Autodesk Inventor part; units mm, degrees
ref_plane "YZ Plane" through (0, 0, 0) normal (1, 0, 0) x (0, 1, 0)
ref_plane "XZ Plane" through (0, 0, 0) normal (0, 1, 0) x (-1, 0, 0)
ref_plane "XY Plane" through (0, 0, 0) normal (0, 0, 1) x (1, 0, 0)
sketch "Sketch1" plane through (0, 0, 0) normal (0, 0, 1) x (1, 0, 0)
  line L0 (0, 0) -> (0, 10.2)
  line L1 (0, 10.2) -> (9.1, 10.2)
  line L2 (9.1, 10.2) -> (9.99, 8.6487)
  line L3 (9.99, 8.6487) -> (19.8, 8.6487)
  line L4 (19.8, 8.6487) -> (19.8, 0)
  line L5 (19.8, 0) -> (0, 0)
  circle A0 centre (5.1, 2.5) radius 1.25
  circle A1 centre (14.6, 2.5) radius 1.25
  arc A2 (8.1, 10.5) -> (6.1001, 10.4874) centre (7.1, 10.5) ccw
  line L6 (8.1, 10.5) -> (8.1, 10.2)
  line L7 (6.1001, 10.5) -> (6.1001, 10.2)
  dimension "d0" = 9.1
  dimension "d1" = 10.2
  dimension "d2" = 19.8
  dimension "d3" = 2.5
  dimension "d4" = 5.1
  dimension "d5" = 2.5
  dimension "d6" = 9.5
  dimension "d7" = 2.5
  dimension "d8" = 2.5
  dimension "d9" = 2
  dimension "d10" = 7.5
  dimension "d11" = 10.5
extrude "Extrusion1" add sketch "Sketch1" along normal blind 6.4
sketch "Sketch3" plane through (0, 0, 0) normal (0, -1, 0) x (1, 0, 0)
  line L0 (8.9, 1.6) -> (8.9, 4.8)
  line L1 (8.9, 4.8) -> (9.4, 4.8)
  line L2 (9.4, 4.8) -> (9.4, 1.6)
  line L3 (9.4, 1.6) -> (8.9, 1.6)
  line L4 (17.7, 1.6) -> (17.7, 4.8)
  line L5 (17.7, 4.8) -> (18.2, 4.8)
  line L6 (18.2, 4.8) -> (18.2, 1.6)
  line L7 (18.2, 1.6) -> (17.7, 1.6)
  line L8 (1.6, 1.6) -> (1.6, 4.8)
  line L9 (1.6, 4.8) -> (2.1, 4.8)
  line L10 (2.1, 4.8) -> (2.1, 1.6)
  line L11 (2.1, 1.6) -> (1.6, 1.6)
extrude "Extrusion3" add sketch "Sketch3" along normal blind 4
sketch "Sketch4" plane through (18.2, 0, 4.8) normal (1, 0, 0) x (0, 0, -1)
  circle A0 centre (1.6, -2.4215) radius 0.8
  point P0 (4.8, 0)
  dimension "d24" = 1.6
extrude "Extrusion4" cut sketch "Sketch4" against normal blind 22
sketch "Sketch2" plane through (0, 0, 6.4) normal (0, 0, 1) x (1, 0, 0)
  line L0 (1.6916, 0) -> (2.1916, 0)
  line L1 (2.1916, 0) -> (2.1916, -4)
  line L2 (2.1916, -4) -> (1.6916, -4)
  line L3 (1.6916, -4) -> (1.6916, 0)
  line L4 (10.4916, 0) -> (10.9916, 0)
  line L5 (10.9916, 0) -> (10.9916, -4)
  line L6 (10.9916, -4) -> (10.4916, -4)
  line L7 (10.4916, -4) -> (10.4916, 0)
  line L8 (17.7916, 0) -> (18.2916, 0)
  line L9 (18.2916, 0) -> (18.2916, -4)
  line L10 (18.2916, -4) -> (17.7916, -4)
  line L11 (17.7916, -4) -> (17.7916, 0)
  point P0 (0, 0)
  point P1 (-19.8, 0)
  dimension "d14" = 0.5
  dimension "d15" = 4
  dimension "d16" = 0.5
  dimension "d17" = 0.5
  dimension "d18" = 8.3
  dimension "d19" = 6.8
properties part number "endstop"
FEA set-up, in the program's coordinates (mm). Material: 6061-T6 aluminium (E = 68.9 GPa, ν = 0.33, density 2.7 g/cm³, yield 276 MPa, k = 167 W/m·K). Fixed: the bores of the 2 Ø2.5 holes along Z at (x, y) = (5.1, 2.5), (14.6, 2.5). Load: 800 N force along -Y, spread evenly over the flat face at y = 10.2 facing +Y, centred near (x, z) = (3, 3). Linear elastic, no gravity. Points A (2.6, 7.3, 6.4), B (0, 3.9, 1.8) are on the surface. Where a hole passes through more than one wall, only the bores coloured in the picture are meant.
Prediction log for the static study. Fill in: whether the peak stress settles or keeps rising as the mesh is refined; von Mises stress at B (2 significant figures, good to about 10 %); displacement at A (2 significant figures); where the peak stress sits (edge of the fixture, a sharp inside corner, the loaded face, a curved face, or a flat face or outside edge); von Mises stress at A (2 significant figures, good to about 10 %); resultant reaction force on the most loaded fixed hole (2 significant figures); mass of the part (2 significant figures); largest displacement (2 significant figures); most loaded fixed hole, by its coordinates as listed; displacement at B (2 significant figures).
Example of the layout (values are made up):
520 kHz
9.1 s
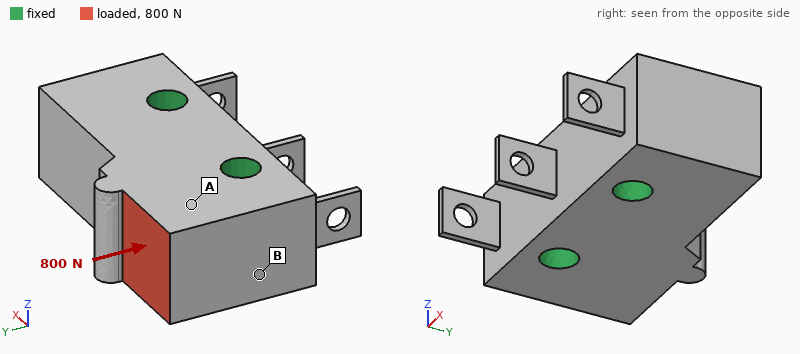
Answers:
keeps rising
8.2 MPa
2.7 µm
edge of the fixture
22 MPa
880 N
3.1 g
4.8 µm
(5.1, 2.5)
2.6 µm
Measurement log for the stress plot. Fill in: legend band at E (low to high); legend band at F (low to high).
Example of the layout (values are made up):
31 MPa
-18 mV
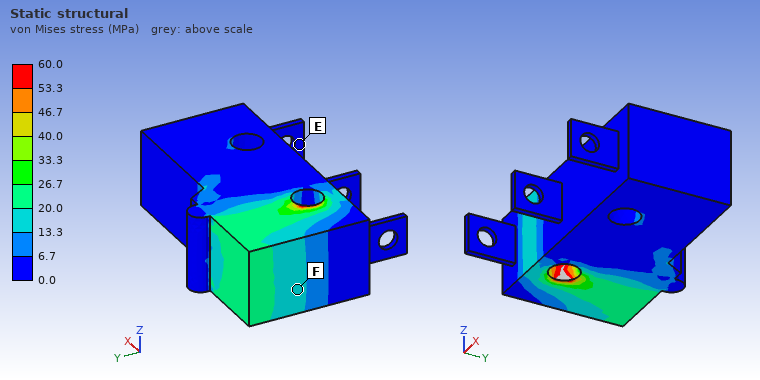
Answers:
0.0 to 6.7 MPa
13.3 to 20.0 MPa
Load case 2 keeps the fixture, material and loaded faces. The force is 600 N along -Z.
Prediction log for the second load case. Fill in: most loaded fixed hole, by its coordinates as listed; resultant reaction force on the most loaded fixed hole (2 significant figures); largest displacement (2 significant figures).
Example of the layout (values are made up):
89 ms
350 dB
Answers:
(5.1, 2.5)
580 N
14 µm
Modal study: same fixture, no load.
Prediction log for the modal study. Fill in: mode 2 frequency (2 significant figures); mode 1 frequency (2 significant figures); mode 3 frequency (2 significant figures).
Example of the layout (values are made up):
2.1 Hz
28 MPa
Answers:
25 kHz
25 kHz
25 kHz
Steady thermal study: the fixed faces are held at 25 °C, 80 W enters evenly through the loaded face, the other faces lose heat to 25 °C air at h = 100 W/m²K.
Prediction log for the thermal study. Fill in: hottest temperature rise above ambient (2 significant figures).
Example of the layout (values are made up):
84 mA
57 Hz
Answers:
74 K
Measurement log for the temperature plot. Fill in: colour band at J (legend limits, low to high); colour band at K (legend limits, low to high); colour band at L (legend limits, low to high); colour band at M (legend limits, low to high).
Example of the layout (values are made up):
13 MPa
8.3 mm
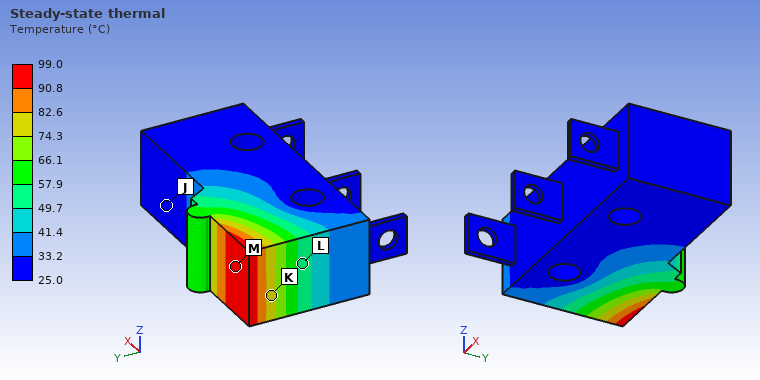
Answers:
25.0 to 33.2 °C
74.3 to 82.6 °C
49.7 to 57.9 °C
90.8 to 99.0 °C
